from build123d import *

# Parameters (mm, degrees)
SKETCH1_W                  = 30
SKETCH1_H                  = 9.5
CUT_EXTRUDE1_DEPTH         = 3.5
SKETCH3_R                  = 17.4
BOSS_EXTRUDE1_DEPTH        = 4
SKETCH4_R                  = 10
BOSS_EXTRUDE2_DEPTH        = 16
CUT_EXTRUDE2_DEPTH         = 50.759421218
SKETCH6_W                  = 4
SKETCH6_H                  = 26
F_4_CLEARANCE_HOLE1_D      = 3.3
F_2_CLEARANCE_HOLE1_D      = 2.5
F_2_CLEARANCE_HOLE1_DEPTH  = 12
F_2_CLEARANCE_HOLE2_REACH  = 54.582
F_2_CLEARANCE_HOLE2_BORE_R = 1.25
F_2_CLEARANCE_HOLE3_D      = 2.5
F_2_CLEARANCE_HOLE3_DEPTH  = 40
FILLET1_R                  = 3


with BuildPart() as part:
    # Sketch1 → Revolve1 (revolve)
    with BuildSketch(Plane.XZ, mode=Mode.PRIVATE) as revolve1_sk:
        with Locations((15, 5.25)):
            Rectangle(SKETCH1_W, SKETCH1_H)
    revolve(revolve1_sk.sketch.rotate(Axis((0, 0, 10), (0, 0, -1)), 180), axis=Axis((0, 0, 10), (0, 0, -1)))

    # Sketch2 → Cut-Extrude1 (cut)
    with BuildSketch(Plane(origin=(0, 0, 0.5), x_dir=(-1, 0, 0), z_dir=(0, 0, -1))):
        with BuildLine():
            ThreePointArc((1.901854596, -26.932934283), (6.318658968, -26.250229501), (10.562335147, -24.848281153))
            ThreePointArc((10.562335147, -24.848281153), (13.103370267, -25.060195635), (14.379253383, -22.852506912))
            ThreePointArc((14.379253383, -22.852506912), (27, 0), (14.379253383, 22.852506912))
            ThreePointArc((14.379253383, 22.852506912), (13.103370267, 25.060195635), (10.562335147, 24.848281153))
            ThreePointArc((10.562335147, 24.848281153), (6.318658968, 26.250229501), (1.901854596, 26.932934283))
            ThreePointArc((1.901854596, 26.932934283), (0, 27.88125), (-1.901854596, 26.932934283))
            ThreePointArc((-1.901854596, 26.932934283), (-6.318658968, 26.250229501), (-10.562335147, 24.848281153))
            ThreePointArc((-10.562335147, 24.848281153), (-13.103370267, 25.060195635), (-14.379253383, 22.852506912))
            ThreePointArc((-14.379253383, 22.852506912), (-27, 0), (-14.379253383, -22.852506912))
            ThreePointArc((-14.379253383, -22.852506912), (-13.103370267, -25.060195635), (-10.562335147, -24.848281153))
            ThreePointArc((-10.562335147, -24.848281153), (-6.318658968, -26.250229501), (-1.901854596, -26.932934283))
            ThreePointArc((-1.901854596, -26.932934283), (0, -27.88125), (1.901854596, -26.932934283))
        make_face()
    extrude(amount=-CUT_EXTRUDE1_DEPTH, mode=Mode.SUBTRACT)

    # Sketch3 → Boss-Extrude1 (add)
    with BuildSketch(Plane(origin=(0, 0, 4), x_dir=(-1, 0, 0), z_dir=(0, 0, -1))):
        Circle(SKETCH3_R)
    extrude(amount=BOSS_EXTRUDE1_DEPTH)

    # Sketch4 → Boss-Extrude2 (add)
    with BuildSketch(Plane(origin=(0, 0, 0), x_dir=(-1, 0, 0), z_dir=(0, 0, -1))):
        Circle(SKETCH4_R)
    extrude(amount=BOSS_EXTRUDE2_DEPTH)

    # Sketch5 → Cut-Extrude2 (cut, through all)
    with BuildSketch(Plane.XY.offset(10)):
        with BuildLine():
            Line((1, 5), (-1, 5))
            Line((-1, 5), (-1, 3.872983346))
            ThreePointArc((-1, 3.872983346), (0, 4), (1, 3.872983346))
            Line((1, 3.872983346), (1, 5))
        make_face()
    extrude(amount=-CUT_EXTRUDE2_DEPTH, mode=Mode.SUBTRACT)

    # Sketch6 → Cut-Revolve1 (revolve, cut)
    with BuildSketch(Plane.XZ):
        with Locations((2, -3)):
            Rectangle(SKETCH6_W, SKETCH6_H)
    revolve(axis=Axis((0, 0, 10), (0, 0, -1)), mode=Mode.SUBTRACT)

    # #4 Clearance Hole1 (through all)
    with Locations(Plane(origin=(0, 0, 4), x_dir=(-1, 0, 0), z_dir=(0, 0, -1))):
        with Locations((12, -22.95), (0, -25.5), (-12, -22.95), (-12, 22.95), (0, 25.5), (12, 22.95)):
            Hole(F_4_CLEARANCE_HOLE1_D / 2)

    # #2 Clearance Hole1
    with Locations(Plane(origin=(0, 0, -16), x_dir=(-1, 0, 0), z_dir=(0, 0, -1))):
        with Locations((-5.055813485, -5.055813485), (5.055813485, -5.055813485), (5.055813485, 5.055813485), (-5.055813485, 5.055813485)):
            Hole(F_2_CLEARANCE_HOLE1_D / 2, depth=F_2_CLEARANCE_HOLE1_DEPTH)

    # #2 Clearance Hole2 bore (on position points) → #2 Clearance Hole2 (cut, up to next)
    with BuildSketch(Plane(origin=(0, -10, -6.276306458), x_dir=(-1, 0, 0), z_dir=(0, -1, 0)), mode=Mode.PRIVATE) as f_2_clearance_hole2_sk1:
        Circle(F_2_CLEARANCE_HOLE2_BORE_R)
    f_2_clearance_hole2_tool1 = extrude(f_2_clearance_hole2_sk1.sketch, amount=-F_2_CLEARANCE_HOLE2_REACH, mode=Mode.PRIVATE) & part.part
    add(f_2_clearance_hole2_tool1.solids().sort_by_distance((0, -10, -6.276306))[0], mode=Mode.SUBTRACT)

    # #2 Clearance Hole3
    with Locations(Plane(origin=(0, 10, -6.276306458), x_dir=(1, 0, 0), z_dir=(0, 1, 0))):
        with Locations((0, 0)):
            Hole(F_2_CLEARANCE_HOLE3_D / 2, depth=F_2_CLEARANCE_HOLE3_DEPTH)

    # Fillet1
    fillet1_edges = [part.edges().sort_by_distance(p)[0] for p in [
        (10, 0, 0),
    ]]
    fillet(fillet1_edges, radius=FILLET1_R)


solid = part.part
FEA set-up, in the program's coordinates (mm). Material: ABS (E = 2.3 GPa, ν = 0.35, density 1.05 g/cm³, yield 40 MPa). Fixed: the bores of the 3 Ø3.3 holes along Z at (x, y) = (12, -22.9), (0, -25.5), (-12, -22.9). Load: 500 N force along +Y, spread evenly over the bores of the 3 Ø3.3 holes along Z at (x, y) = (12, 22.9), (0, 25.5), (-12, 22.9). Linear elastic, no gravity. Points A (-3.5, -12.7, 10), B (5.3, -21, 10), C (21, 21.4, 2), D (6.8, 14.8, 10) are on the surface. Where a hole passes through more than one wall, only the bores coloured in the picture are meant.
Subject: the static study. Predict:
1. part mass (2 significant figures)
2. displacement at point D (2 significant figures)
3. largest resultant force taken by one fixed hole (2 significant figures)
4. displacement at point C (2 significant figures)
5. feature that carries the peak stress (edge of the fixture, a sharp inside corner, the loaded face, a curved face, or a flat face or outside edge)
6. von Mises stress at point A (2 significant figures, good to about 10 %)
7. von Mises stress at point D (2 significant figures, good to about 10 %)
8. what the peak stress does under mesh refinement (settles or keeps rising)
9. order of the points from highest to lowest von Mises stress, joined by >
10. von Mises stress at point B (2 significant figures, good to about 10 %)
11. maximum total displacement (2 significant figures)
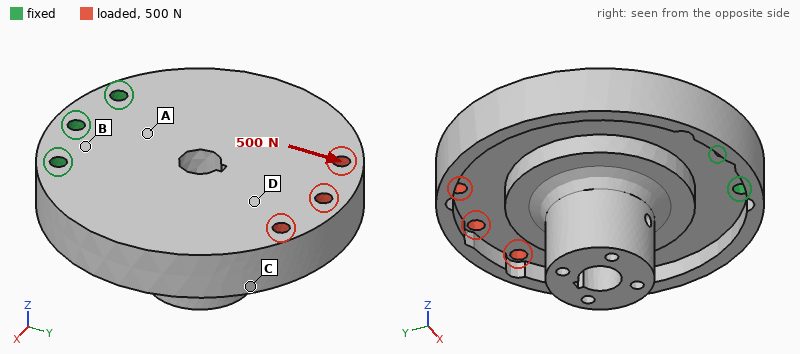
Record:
27 g
0.069 mm
190 N
0.064 mm
edge of the fixture
2.0 MPa
2.5 MPa
keeps rising
D > A > B > C
1.1 MPa
0.12 mm
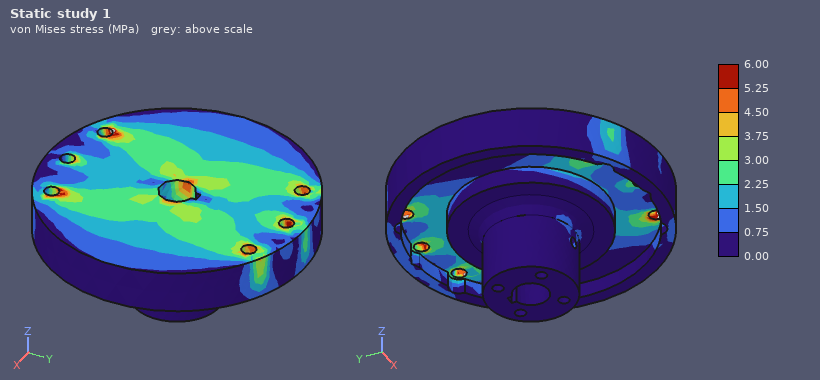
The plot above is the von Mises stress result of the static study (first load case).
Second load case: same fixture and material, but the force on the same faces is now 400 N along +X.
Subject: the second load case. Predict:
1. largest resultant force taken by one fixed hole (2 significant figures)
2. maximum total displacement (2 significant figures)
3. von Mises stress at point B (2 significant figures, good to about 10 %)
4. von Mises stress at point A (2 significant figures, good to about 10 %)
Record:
730 N
0.36 mm
4.6 MPa
7.3 MPa
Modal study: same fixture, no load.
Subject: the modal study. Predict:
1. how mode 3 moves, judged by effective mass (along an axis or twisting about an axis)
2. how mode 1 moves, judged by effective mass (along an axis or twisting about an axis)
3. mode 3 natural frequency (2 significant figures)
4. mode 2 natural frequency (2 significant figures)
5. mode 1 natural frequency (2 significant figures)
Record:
along X
along Z
1800 Hz
1500 Hz
520 Hz
